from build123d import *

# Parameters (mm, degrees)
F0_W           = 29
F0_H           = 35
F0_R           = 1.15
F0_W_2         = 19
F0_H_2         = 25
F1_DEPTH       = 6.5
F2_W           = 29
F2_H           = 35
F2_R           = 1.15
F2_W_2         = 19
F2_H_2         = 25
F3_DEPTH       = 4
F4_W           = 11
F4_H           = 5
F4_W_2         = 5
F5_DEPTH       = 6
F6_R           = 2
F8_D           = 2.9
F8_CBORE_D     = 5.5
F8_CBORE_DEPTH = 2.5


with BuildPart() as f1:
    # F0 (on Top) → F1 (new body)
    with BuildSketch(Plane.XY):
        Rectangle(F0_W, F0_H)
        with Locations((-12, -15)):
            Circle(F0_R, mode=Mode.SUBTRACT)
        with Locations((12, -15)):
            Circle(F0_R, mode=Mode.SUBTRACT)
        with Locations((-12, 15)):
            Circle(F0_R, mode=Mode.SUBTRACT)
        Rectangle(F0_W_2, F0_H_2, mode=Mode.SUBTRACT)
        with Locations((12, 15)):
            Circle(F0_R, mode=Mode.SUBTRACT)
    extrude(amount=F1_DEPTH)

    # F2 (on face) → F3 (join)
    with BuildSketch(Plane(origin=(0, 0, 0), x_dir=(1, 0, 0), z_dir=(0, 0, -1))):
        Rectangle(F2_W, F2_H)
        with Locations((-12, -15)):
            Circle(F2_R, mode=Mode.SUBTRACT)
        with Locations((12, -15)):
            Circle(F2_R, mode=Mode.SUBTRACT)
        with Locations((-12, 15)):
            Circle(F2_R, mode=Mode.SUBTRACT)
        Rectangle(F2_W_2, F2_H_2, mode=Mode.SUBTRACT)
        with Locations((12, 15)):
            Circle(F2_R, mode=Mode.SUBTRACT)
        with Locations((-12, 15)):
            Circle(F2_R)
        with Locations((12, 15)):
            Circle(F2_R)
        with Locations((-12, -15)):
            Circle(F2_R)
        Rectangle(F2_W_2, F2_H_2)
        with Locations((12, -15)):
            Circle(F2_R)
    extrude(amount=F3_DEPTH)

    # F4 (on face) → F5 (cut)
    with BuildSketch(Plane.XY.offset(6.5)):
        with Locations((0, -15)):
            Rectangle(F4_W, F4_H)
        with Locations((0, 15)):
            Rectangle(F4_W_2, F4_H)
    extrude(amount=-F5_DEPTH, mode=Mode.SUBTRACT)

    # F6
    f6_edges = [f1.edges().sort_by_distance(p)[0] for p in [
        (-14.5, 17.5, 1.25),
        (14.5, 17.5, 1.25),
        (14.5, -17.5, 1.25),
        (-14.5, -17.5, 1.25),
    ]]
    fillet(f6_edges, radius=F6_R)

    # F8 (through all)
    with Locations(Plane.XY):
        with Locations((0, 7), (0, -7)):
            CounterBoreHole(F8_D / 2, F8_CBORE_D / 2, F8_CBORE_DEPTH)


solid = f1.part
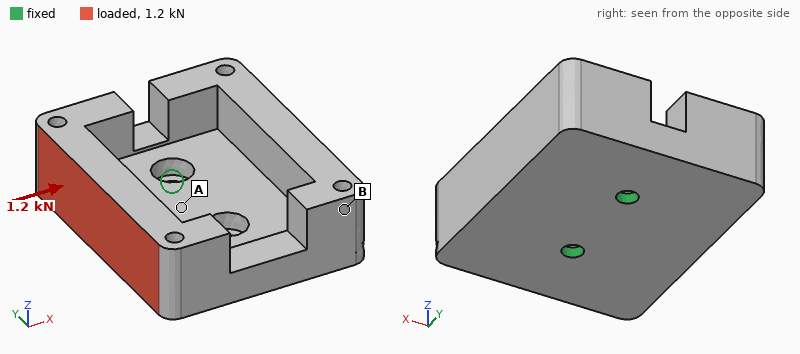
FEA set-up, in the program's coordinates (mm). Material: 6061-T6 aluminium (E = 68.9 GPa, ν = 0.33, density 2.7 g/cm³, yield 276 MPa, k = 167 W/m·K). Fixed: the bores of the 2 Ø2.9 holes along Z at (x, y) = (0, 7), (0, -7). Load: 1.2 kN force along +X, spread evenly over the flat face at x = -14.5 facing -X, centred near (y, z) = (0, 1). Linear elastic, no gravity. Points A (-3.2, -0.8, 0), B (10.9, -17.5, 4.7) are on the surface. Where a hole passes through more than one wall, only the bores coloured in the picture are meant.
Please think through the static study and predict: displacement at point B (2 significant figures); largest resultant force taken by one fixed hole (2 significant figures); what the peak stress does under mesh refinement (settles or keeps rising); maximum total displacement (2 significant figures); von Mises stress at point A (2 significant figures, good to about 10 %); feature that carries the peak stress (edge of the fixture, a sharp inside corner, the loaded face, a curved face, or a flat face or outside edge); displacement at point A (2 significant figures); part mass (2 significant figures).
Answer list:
0.081 mm
600 N
keeps rising
0.14 mm
54 MPa
edge of the fixture
0.030 mm
18 g
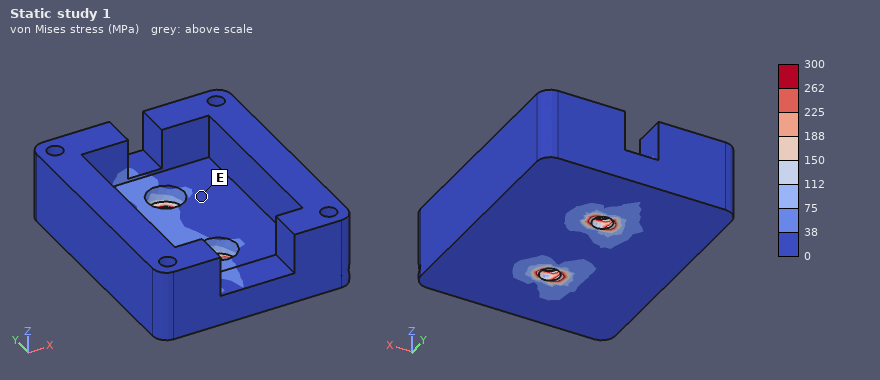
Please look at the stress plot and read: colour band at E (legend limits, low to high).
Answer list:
0 to 38 MPa
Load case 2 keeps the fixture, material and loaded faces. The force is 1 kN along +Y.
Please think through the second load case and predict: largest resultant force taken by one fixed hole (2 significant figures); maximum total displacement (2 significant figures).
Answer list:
1.1 kN
26 µm
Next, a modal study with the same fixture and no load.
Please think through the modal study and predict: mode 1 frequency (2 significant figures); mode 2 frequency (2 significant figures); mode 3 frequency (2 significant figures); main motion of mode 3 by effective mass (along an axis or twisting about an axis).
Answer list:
3200 Hz
8400 Hz
9100 Hz
along Z
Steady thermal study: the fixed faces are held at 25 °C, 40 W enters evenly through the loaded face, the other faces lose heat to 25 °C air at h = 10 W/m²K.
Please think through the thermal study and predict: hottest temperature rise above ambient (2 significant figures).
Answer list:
33 K
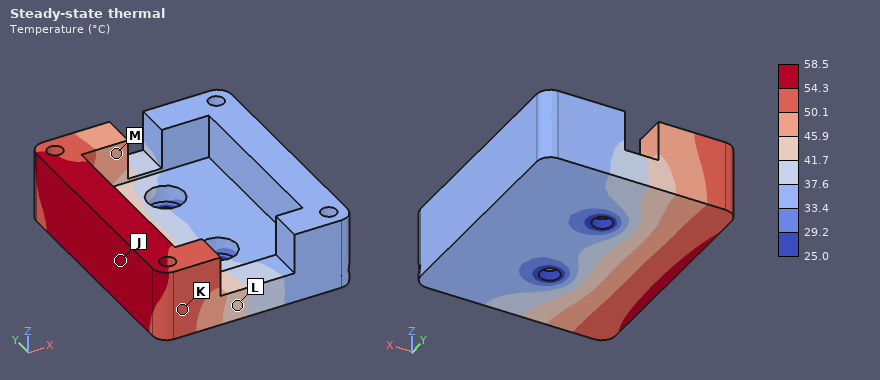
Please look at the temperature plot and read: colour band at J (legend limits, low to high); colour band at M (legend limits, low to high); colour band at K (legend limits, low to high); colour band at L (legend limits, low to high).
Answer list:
54.3 to 58.5 °C
45.9 to 50.1 °C
50.1 to 54.3 °C
41.7 to 45.9 °C
